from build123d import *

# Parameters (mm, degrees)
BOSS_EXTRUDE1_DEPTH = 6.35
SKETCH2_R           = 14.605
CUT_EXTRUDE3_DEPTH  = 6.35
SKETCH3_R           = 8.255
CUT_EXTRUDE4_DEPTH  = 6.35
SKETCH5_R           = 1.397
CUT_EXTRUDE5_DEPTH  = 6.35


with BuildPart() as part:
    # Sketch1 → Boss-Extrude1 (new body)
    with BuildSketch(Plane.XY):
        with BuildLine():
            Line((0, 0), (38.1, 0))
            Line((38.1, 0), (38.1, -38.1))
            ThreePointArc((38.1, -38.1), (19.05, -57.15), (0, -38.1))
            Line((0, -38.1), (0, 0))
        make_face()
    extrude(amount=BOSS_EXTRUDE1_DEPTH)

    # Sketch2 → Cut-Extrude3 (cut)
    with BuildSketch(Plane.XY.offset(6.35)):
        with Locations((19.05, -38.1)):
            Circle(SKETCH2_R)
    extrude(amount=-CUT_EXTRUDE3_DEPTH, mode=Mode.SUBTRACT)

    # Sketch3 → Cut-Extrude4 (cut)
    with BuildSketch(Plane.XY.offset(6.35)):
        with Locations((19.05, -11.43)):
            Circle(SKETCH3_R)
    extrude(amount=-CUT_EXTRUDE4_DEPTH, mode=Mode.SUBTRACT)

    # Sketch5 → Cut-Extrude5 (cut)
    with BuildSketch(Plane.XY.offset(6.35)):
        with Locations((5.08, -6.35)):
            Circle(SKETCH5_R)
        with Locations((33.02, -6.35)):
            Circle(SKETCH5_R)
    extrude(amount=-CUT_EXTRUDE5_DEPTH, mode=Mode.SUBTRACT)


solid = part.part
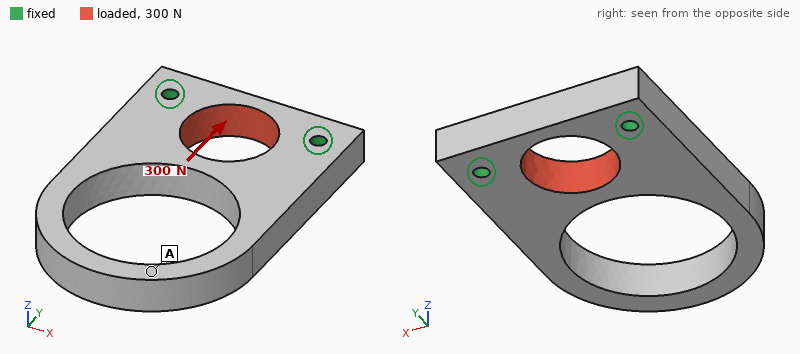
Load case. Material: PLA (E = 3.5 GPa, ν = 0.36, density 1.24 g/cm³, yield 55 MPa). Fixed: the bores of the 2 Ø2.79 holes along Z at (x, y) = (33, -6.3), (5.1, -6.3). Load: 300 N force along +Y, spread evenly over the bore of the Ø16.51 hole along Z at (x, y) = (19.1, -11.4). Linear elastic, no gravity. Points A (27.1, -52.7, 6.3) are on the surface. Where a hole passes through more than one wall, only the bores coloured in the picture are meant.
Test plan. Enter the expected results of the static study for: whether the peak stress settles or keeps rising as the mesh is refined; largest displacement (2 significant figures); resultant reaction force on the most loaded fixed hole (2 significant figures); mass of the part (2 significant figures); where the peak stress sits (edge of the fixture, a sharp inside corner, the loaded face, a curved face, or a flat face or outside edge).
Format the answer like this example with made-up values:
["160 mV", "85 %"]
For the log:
["keeps rising", "24 µm", "150 N", "8.9 g", "edge of the fixture"]
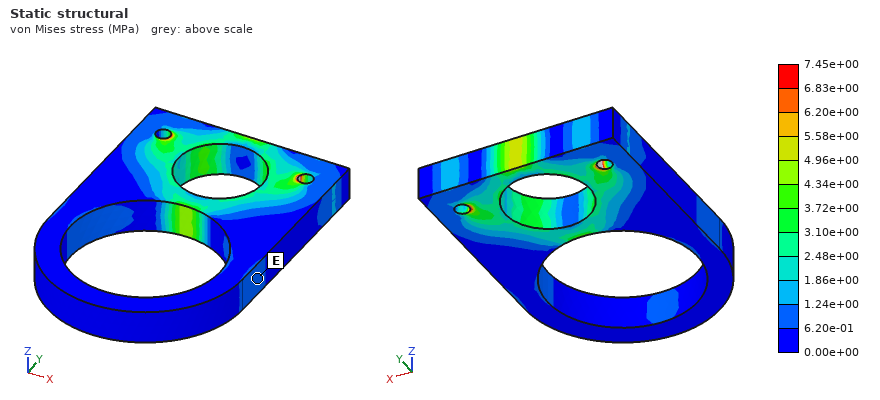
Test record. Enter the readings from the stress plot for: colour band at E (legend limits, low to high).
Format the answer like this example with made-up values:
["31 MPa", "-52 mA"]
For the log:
["6.20e-01 to 1.24e+00 MPa"]
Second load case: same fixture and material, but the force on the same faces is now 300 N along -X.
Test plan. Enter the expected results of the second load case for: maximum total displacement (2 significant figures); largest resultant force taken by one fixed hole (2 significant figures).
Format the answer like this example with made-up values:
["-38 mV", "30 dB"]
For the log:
["58 µm", "150 N"]
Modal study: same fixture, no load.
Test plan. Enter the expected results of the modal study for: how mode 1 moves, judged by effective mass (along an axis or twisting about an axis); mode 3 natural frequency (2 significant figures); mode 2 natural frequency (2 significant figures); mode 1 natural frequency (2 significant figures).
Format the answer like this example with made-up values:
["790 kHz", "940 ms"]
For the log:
["along Z", "1800 Hz", "1800 Hz", "780 Hz"]
